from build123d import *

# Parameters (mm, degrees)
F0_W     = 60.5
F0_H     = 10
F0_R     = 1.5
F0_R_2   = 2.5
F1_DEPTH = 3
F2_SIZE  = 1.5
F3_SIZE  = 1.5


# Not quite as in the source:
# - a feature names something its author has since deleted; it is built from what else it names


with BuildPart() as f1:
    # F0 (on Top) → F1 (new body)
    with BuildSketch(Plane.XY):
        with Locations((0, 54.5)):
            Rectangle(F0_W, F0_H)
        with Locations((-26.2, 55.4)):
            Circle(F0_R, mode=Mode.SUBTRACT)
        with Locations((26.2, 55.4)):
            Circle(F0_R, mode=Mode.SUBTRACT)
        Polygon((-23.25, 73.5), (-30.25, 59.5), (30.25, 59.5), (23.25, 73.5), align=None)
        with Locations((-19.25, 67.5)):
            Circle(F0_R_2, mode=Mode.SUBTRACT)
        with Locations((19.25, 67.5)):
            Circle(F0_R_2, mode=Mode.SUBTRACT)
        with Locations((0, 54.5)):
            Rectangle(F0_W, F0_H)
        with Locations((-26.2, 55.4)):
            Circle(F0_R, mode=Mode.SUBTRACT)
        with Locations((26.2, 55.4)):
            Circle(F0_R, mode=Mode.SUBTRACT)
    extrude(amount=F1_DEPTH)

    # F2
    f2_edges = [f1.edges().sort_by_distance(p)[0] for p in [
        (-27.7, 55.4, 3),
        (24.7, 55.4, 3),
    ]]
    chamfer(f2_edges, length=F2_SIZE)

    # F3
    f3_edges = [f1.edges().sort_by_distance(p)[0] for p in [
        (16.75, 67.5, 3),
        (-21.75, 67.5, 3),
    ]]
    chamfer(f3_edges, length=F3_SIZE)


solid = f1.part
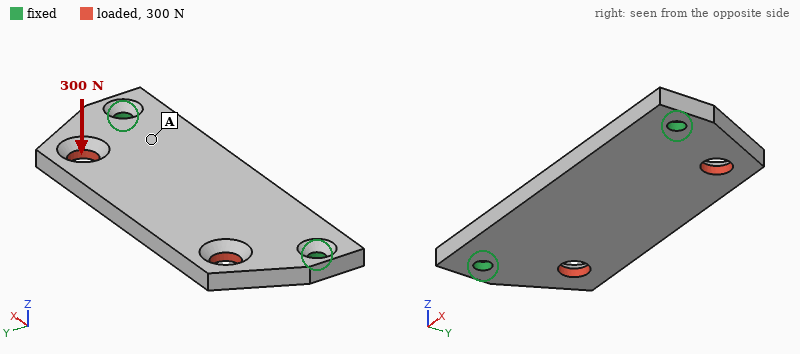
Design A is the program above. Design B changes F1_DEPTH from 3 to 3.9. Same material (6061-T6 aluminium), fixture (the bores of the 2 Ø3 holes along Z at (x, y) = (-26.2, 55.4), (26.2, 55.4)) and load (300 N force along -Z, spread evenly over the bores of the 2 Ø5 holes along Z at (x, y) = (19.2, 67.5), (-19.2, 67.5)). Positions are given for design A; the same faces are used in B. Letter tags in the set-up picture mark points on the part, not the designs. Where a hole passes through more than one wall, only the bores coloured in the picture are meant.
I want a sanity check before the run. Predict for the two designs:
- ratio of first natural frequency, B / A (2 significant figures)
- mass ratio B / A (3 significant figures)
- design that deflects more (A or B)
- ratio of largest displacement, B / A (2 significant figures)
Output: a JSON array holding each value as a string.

["1.3", "1.31", "A", "0.45"]
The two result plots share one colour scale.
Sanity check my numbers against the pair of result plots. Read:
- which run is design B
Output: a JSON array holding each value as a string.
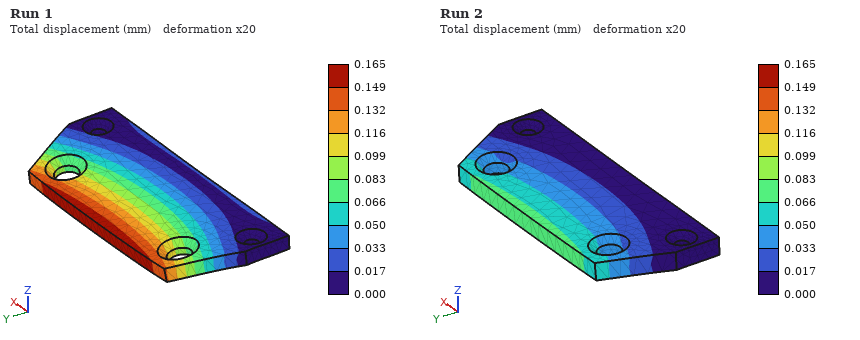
["Run 2"]
